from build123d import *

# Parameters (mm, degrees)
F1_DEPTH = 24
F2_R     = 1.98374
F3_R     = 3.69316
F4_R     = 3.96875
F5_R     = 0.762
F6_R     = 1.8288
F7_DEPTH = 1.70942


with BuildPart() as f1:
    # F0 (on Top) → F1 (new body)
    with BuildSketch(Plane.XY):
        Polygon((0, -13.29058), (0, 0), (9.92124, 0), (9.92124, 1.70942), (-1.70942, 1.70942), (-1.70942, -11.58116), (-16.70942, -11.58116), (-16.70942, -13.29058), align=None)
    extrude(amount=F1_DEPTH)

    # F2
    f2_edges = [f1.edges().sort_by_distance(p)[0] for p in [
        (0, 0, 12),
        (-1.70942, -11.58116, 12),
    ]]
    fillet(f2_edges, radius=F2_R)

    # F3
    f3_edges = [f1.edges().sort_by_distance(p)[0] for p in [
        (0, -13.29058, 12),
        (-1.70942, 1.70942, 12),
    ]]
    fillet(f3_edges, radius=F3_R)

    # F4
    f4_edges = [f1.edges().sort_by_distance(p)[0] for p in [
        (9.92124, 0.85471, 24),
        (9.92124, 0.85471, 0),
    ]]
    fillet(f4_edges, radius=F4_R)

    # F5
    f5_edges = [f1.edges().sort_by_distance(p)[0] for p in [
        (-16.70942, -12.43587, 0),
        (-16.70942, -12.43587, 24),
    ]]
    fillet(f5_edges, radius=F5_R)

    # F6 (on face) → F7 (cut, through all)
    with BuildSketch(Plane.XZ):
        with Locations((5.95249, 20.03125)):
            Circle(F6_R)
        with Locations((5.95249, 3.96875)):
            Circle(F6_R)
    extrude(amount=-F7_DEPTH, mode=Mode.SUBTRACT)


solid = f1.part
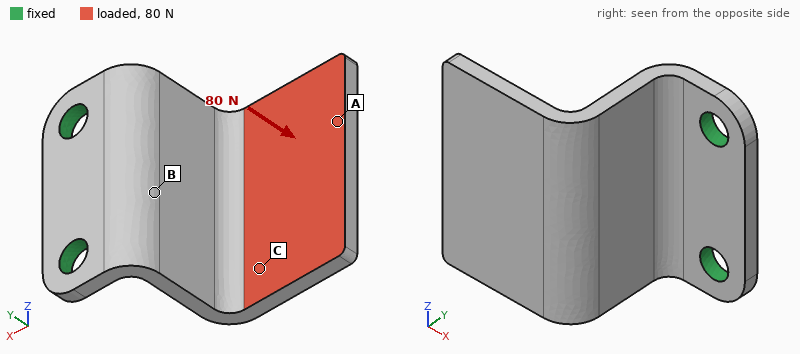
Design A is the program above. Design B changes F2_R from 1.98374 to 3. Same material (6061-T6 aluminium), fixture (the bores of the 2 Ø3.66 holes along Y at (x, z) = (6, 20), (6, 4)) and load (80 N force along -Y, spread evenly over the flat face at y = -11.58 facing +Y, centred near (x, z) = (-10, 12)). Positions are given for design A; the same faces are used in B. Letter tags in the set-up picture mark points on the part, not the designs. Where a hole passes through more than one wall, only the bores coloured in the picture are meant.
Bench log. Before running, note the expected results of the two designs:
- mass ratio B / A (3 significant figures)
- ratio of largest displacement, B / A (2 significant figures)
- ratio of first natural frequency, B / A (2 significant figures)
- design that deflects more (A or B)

1.04
0.87
1.1
A
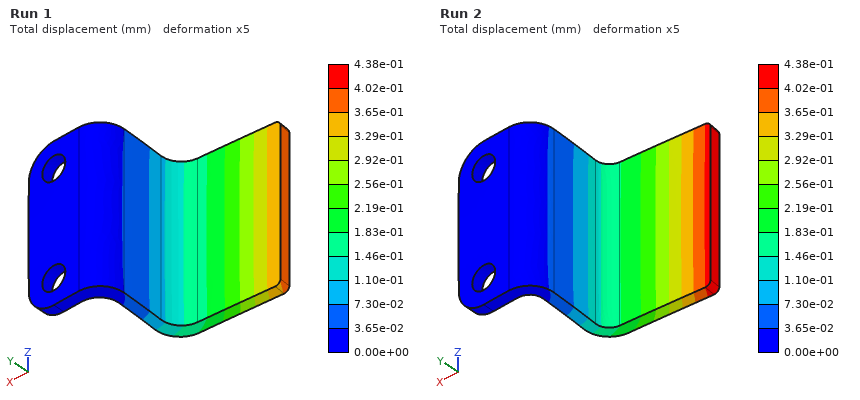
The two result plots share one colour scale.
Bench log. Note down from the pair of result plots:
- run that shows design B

Run 1
